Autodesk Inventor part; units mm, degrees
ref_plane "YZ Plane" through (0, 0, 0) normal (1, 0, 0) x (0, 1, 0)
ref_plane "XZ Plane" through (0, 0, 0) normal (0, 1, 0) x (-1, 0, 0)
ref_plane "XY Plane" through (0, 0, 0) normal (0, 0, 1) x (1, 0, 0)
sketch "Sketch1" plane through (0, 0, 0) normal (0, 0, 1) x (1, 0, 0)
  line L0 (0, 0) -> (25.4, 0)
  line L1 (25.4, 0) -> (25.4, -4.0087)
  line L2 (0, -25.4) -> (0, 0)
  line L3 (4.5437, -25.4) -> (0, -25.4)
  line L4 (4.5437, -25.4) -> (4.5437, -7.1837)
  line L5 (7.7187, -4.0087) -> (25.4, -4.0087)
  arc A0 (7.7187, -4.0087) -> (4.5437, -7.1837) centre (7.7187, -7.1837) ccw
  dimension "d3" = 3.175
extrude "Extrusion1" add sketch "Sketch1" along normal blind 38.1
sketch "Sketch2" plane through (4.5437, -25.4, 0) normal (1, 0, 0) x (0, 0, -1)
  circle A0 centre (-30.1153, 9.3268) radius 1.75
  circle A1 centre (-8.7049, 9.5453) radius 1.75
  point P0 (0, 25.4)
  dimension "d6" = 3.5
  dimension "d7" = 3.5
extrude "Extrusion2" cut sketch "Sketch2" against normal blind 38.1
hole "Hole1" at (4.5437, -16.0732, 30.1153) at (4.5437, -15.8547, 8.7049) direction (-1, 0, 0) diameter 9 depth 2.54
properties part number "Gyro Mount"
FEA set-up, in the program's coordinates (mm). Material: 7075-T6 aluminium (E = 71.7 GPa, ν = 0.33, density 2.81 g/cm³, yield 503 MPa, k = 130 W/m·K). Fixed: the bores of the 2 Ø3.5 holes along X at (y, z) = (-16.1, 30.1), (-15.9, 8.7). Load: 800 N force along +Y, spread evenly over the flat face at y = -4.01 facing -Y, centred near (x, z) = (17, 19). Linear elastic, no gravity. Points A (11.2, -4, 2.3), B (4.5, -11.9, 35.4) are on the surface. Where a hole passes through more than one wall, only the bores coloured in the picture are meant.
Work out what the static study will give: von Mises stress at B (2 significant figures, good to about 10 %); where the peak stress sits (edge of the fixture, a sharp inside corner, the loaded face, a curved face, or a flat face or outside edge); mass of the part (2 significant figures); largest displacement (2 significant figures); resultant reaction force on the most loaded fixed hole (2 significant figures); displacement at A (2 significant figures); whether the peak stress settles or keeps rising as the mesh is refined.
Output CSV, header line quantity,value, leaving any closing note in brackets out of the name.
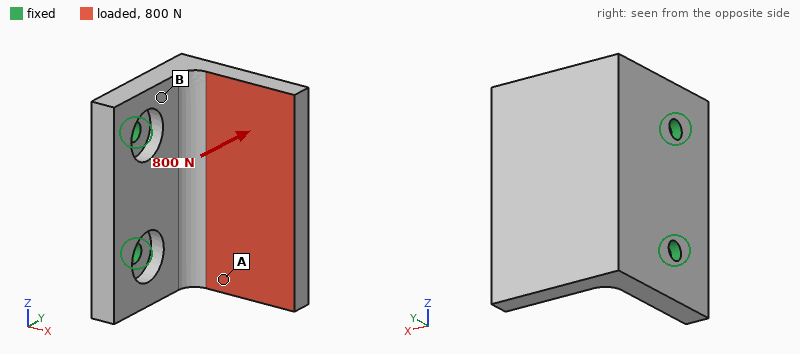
quantity,value
von Mises stress at B,130 MPa
where the peak stress sits,edge of the fixture
mass of the part,21 g
largest displacement,0.47 mm
resultant reaction force on the most loaded fixed hole,410 N
displacement at A,0.20 mm
whether the peak stress settles or keeps rising as the mesh is refined,keeps rising
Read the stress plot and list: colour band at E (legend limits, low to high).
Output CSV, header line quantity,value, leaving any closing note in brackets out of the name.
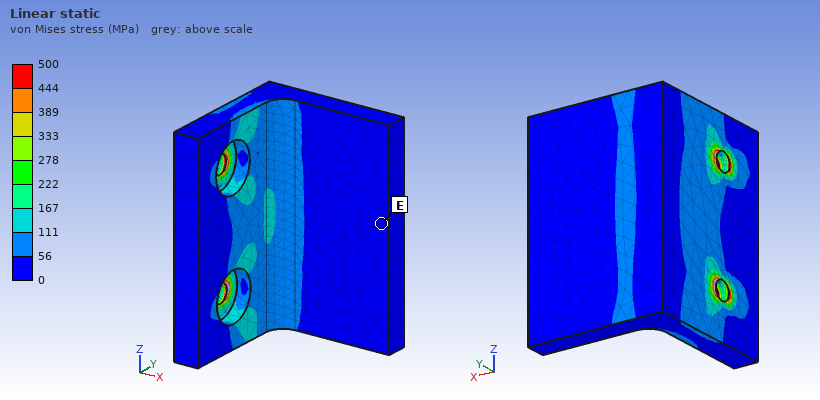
quantity,value
colour band at E,0 to 56 MPa
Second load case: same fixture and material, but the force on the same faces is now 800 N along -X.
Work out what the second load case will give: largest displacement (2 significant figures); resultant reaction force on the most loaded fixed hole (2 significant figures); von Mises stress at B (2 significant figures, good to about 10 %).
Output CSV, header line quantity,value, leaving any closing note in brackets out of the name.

quantity,value
largest displacement,0.23 mm
resultant reaction force on the most loaded fixed hole,420 N
von Mises stress at B,71 MPa
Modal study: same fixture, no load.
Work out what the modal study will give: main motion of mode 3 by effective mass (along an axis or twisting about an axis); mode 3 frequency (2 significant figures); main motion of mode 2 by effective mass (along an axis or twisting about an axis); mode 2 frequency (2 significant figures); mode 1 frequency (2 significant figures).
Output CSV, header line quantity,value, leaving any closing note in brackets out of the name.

quantity,value
main motion of mode 3 by effective mass,along X
mode 3 frequency,8800 Hz
main motion of mode 2 by effective mass,along Z
mode 2 frequency,5300 Hz
mode 1 frequency,2400 Hz
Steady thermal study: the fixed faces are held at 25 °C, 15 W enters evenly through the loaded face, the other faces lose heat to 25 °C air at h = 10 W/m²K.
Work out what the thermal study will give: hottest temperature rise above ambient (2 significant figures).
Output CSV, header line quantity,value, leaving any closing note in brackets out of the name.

quantity,value
hottest temperature rise above ambient,22 K
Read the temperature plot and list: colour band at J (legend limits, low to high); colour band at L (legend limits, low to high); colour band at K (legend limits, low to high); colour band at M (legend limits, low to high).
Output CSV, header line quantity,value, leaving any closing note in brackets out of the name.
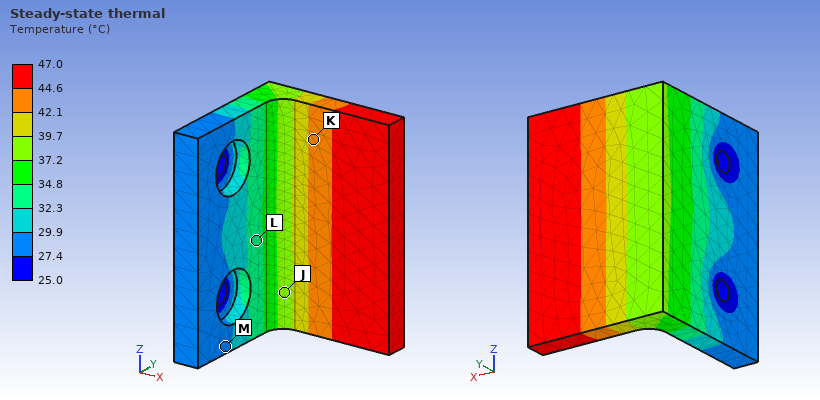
quantity,value
colour band at J,37.2 to 39.7 °C
colour band at L,32.3 to 34.8 °C
colour band at K,42.1 to 44.6 °C
colour band at M,27.4 to 29.9 °C
